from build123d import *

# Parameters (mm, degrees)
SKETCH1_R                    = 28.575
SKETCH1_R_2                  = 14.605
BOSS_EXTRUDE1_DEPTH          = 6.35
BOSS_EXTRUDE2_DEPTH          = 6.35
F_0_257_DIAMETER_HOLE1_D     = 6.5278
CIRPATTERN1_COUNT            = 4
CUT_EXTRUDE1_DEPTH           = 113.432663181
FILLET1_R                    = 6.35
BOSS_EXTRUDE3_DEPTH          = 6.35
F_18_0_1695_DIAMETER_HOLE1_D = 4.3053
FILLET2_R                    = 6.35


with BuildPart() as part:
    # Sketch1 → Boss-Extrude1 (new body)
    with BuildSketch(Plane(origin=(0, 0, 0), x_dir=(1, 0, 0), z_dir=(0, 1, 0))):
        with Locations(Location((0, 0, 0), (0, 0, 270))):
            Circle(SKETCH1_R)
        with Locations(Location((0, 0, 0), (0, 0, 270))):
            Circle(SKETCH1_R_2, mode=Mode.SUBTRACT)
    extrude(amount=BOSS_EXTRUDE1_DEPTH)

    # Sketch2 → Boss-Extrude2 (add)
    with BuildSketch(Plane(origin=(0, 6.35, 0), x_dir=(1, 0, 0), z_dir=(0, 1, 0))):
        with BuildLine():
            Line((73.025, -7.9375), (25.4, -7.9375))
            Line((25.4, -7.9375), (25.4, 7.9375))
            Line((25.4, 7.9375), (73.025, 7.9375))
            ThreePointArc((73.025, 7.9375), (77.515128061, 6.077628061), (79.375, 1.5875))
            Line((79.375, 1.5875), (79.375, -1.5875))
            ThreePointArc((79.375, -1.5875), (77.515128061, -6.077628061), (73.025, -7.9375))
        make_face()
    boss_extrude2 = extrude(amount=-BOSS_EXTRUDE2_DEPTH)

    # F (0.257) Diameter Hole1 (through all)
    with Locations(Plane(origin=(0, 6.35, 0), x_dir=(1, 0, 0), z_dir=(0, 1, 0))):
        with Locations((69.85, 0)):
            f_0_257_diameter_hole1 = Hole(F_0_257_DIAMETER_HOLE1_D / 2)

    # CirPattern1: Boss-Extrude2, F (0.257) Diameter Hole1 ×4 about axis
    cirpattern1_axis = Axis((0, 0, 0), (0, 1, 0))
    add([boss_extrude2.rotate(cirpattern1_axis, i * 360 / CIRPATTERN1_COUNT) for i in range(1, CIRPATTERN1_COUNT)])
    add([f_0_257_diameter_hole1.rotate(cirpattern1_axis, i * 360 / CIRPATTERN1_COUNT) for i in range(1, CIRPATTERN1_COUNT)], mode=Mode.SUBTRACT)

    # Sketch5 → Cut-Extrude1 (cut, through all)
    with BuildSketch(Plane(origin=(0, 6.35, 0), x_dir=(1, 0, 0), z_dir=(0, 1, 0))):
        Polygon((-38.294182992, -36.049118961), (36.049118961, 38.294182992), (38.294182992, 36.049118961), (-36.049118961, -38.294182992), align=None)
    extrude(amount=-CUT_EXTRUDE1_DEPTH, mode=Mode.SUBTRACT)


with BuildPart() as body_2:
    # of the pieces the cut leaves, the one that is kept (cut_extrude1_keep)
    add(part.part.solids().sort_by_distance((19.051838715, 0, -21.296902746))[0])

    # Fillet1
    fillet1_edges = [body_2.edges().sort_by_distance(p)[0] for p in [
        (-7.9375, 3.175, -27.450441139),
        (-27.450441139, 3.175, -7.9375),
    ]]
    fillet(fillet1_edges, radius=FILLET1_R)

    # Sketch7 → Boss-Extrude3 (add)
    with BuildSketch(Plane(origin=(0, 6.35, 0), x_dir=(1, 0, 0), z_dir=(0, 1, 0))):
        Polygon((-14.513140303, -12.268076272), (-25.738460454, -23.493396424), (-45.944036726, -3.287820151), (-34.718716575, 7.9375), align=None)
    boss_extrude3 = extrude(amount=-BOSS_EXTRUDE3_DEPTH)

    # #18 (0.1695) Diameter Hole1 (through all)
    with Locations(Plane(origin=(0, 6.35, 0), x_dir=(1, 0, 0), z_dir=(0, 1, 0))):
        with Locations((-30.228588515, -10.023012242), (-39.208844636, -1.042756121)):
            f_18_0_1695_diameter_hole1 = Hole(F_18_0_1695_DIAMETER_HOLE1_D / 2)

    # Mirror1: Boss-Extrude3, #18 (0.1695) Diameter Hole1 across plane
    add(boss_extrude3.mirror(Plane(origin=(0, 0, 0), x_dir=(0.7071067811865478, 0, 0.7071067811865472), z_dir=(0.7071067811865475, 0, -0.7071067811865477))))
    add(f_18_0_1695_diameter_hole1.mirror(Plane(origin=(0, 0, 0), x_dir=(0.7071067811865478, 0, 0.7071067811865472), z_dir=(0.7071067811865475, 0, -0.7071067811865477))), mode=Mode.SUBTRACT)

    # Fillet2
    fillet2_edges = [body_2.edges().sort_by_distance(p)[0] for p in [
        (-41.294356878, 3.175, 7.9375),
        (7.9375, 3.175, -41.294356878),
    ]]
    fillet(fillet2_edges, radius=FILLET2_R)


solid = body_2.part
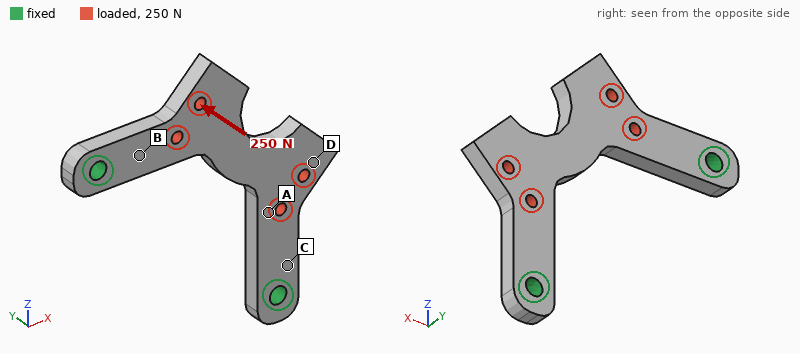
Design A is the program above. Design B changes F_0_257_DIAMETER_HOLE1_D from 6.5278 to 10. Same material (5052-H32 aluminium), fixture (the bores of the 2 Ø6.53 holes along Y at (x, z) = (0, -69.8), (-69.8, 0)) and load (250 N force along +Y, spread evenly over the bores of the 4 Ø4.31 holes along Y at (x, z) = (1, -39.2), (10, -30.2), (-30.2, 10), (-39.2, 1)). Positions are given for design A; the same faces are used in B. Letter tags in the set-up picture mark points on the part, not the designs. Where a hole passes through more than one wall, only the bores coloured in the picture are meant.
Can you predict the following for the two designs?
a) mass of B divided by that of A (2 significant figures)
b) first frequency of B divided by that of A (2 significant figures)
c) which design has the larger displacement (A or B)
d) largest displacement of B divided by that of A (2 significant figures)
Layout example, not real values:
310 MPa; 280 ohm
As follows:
0.97; 1.1; A; 0.86
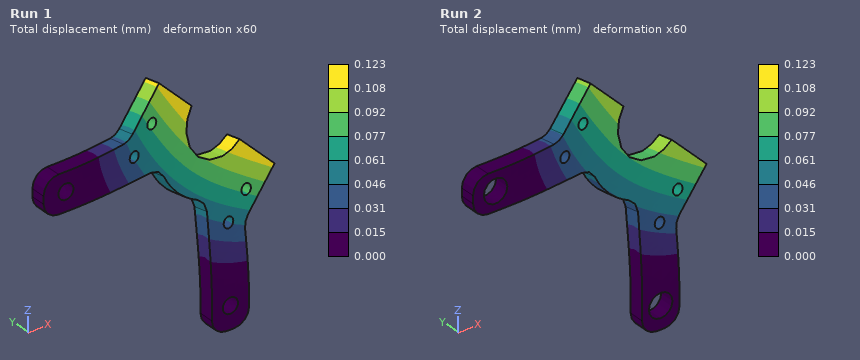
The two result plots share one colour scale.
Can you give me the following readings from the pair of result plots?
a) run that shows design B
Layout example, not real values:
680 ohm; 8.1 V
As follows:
Run 2
